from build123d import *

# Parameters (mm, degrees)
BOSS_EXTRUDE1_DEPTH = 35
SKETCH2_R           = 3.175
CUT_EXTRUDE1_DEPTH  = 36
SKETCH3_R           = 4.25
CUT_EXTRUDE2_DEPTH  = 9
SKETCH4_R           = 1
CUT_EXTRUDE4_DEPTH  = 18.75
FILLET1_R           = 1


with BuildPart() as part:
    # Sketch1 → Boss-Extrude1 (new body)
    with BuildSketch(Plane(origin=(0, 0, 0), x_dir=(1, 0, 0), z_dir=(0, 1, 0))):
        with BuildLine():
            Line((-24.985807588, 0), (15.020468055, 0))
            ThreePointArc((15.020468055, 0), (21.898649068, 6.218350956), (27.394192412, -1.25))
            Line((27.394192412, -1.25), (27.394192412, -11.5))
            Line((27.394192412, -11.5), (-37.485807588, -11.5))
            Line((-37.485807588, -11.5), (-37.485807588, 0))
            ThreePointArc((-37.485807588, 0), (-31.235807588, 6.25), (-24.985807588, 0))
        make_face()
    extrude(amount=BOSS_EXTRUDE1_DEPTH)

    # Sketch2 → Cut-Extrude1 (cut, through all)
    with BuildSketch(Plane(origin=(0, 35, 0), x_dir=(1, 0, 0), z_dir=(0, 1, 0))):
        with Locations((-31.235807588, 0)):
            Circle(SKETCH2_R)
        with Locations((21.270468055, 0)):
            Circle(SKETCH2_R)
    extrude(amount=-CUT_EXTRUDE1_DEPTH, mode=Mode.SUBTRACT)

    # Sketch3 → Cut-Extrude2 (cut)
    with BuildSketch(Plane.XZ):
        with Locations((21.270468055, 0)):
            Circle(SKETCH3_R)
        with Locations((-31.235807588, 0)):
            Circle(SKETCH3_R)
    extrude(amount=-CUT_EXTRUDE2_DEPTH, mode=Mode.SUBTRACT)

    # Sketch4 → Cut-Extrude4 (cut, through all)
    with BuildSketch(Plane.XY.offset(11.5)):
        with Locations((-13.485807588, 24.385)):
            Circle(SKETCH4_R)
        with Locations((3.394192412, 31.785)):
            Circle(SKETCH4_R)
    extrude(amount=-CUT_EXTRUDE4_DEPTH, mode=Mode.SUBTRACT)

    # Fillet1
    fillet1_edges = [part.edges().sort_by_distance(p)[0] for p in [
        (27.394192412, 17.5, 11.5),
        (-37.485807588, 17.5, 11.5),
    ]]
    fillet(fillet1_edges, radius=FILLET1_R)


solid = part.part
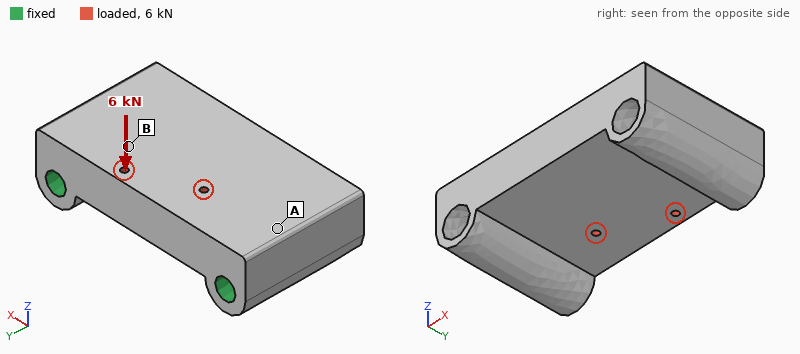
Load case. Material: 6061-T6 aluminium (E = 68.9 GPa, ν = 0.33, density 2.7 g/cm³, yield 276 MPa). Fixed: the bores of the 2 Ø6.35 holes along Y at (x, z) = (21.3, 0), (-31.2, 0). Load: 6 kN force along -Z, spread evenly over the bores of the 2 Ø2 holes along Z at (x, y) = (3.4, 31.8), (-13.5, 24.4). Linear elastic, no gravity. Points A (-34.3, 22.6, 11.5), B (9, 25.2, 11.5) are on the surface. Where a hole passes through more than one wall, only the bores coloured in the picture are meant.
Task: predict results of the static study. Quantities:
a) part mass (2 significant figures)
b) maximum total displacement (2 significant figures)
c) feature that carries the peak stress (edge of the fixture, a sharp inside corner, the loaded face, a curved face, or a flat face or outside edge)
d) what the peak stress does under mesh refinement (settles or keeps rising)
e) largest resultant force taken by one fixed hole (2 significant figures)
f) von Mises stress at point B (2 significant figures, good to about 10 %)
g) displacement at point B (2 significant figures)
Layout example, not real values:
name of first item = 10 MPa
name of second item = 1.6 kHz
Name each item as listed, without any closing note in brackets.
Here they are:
part mass = 75 g
maximum total displacement = 34 µm
feature that carries the peak stress = a sharp inside corner
what the peak stress does under mesh refinement = keeps rising
largest resultant force taken by one fixed hole = 3.7 kN
von Mises stress at point B = 34 MPa
displacement at point B = 14 µm
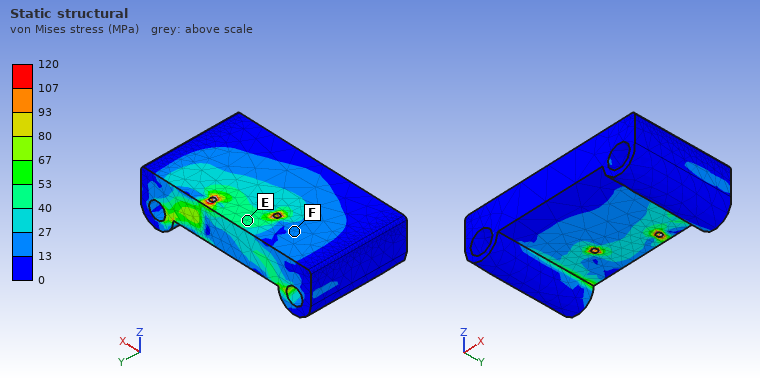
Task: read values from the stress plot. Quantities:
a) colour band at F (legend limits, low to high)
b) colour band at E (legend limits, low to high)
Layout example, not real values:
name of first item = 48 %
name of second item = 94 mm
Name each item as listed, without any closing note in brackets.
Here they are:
colour band at F = 13 to 27 MPa
colour band at E = 40 to 53 MPa
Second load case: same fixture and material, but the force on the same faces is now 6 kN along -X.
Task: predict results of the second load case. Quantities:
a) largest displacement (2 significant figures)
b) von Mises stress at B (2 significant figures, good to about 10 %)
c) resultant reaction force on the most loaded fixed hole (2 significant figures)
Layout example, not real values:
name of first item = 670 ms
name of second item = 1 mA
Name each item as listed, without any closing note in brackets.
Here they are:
largest displacement = 7.0 µm
von Mises stress at B = 6.9 MPa
resultant reaction force on the most loaded fixed hole = 3.1 kN
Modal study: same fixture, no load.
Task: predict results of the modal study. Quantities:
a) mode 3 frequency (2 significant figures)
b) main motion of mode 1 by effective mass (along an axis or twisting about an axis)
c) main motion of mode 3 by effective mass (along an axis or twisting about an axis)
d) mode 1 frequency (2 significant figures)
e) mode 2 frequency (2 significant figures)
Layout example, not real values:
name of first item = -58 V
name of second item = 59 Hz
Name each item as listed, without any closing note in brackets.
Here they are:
mode 3 frequency = 23 kHz
main motion of mode 1 by effective mass = along Z
main motion of mode 3 by effective mass = along Y
mode 1 frequency = 16 kHz
mode 2 frequency = 21 kHz
